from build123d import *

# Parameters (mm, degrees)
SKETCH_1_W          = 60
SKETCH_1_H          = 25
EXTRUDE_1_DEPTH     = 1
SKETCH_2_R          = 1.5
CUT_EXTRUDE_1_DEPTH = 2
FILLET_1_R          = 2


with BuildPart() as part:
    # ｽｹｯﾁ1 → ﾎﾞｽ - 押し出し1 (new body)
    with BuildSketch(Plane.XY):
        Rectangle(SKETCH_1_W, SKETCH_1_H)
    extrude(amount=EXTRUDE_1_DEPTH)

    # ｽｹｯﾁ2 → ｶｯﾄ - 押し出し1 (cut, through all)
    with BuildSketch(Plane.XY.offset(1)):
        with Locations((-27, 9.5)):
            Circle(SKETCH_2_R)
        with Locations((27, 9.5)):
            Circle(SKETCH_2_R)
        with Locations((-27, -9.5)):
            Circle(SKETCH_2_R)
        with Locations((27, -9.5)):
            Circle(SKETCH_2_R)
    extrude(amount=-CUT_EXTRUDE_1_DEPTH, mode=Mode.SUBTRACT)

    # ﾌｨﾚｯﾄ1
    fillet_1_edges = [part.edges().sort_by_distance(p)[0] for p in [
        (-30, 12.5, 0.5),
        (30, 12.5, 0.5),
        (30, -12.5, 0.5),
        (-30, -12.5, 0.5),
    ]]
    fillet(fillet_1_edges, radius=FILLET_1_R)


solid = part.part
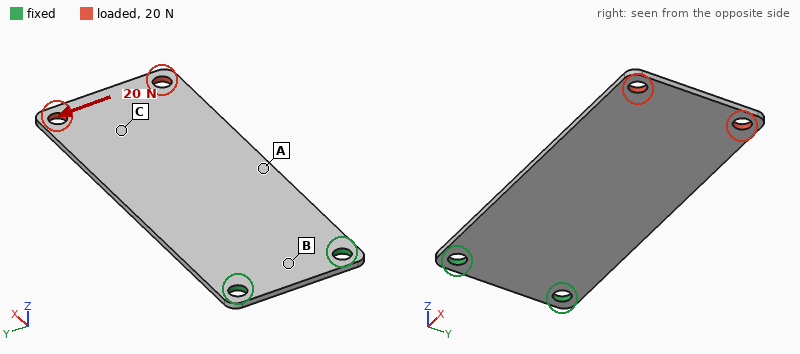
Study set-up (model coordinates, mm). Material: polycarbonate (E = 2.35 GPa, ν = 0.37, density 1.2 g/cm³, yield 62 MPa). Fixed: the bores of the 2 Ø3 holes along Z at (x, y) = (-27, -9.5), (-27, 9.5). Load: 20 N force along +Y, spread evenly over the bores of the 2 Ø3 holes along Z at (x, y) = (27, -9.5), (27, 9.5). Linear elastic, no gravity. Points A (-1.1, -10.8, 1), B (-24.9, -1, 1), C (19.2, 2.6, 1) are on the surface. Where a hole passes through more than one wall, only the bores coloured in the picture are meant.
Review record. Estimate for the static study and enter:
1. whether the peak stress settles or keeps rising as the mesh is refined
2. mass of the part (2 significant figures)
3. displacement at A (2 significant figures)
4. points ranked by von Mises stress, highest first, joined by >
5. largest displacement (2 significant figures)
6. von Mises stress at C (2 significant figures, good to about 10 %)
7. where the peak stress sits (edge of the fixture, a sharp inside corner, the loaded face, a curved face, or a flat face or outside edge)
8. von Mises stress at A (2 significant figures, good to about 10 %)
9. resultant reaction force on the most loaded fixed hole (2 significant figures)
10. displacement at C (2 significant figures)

keeps rising
1.8 g
0.15 mm
A > C > B
0.44 mm
2.0 MPa
edge of the fixture
4.7 MPa
55 N
0.32 mm
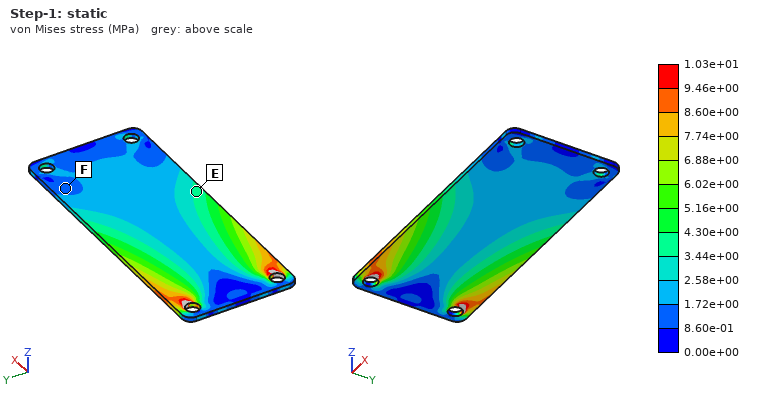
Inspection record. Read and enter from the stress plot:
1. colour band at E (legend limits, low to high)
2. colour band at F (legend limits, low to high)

3.44e+00 to 4.30e+00 MPa
8.60e-01 to 1.72e+00 MPa
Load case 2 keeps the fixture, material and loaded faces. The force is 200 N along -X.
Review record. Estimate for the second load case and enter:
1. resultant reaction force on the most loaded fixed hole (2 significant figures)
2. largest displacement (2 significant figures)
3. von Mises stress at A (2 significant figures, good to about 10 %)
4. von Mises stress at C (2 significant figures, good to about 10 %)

100 N
0.26 mm
8.0 MPa
5.1 MPa
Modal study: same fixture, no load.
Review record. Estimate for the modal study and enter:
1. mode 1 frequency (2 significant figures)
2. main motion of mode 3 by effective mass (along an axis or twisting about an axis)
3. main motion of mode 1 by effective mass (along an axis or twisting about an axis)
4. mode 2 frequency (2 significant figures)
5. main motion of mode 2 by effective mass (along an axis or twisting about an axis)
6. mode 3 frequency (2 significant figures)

72 Hz
along Z
along Z
350 Hz
twisting about X
450 Hz
